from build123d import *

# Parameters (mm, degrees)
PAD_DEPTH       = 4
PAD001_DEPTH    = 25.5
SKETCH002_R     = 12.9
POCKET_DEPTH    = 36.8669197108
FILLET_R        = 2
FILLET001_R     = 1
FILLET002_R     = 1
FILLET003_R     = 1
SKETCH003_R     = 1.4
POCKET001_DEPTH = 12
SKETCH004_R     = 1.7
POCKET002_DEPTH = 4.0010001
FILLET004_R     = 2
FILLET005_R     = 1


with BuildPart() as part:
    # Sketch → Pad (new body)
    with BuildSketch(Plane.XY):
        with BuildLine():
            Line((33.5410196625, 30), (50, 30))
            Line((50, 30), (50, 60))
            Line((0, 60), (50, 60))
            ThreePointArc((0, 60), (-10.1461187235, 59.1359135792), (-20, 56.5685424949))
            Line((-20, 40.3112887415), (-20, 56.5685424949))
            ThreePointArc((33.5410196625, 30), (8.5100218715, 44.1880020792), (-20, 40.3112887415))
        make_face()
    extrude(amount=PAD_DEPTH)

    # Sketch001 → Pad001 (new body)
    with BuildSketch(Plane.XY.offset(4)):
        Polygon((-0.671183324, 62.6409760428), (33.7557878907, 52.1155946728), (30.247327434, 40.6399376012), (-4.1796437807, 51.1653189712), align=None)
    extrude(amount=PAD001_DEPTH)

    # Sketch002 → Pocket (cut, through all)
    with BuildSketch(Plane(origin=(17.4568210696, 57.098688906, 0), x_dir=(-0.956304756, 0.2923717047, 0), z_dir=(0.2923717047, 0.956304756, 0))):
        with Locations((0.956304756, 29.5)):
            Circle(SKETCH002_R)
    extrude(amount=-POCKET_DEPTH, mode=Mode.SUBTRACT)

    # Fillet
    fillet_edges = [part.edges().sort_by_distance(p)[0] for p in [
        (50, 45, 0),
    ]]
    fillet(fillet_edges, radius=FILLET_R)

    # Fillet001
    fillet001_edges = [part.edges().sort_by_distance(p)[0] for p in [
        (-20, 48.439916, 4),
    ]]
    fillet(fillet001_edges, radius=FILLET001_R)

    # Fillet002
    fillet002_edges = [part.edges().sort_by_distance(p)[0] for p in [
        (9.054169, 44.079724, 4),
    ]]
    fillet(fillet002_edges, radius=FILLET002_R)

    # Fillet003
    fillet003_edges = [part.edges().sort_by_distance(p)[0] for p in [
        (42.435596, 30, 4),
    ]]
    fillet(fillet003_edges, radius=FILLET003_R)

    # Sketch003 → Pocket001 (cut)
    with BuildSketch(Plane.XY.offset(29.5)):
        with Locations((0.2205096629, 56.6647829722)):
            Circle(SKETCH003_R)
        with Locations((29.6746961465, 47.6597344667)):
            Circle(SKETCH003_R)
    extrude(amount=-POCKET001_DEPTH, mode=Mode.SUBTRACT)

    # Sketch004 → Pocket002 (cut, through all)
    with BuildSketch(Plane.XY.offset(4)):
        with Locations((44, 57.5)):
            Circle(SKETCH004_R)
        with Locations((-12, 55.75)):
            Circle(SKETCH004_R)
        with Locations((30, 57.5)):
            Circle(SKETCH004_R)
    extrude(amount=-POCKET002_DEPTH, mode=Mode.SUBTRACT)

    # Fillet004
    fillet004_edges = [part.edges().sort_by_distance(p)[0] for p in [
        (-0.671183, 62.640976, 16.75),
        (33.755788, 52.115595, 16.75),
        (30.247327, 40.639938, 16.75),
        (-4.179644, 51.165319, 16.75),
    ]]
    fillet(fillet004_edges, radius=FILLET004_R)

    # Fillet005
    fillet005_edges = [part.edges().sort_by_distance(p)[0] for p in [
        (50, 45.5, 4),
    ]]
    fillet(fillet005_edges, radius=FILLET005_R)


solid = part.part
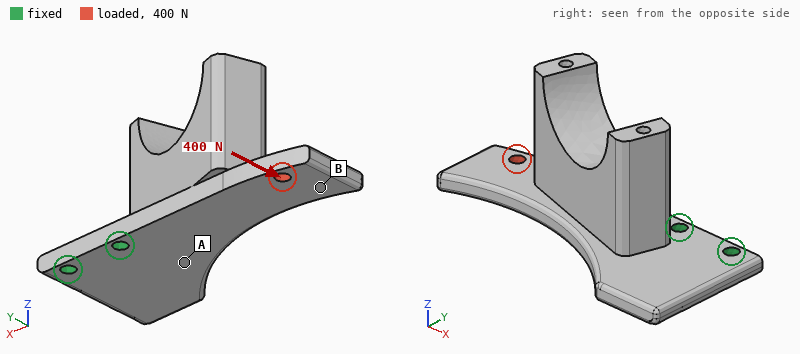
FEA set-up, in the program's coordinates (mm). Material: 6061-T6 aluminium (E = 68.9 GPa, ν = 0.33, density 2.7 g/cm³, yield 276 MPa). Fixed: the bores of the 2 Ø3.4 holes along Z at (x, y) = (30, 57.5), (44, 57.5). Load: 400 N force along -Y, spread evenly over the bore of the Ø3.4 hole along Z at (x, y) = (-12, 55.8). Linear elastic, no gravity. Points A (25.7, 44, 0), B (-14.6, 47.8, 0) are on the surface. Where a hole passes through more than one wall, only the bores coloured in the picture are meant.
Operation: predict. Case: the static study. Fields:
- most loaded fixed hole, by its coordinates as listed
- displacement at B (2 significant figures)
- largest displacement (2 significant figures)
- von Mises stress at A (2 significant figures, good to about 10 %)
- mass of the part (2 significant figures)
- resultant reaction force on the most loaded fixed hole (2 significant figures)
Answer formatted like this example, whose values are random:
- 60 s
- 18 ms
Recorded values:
- (30, 57.5)
- 0.098 mm
- 0.12 mm
- 22 MPa
- 36 g
- 1.4 kN
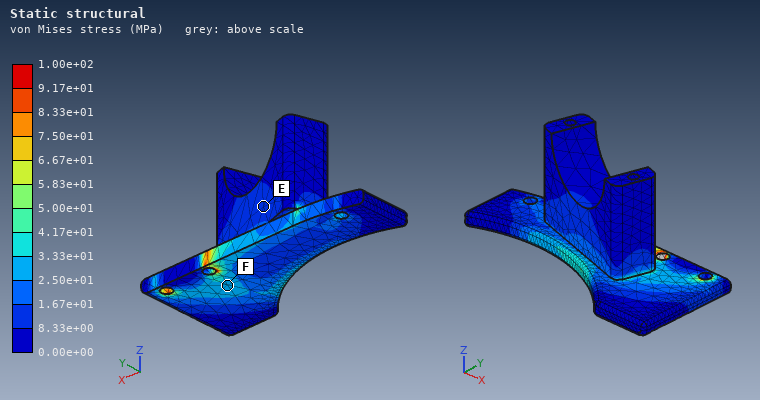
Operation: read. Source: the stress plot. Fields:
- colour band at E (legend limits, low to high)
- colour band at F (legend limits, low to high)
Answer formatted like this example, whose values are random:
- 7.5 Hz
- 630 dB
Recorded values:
- 8.33e+00 to 1.67e+01 MPa
- 2.50e+01 to 3.33e+01 MPa
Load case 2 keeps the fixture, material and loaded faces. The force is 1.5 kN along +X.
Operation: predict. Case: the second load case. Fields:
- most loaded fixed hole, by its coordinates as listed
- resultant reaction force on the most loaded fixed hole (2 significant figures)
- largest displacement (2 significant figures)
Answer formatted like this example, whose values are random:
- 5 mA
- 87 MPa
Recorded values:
- (30, 57.5)
- 1.3 kN
- 54 µm
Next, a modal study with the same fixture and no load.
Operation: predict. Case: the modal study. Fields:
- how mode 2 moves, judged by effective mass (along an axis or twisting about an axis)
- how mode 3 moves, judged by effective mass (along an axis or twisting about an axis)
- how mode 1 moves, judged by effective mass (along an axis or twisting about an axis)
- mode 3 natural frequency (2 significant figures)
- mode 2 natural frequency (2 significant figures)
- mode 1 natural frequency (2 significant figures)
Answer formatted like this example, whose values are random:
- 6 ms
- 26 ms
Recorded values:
- along Y
- along Y
- along Z
- 4500 Hz
- 2600 Hz
- 1600 Hz
